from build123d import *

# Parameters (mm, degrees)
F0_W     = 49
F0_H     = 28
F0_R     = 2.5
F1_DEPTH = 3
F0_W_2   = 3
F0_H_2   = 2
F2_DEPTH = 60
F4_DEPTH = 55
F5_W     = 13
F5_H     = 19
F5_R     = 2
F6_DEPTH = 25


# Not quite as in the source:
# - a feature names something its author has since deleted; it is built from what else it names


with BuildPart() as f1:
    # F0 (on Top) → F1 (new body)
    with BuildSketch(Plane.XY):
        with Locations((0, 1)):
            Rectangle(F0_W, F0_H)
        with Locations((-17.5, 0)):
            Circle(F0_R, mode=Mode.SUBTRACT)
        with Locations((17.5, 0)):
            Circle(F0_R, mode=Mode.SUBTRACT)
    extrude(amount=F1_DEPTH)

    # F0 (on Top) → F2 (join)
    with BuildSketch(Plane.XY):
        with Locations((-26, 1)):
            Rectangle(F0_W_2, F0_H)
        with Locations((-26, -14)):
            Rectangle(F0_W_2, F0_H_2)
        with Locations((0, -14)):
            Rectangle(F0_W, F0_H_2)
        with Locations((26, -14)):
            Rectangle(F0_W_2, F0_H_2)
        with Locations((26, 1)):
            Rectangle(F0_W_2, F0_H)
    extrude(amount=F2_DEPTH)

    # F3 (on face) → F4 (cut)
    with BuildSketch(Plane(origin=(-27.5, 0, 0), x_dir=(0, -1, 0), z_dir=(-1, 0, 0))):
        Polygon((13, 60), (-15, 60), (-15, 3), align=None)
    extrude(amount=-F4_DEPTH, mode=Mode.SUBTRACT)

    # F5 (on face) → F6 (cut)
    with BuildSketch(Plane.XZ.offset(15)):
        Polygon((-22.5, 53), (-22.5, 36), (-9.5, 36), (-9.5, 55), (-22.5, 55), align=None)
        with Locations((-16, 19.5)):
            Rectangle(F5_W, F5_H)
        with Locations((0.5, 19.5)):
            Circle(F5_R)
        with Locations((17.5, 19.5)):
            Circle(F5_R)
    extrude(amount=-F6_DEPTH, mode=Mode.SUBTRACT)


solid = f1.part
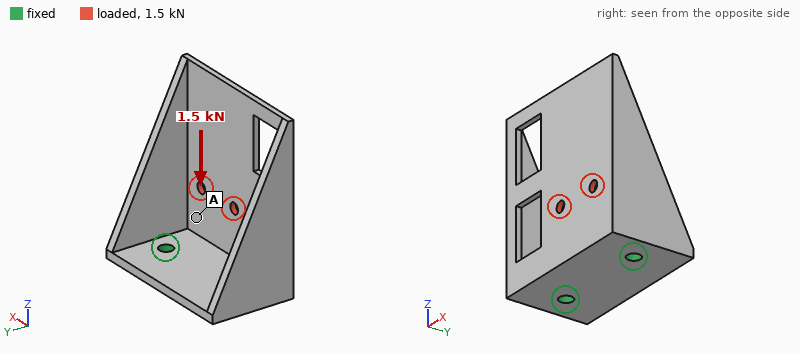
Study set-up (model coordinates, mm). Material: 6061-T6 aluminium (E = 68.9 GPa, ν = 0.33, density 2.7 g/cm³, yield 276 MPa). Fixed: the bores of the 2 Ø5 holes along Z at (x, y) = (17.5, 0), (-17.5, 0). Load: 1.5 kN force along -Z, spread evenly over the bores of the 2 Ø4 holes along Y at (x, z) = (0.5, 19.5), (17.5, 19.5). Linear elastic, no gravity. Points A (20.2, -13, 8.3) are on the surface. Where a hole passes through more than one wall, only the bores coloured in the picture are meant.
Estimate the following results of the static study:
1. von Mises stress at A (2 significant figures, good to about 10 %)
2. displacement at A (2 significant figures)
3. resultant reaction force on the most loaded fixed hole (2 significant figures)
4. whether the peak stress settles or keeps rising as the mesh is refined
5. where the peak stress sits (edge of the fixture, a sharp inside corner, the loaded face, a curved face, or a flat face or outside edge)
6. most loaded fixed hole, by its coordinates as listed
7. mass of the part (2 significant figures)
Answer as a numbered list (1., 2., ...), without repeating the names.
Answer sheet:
1. 29 MPa
2. 0.14 mm
3. 1.1 kN
4. keeps rising
5. edge of the fixture
6. (17.5, 0)
7. 40 g
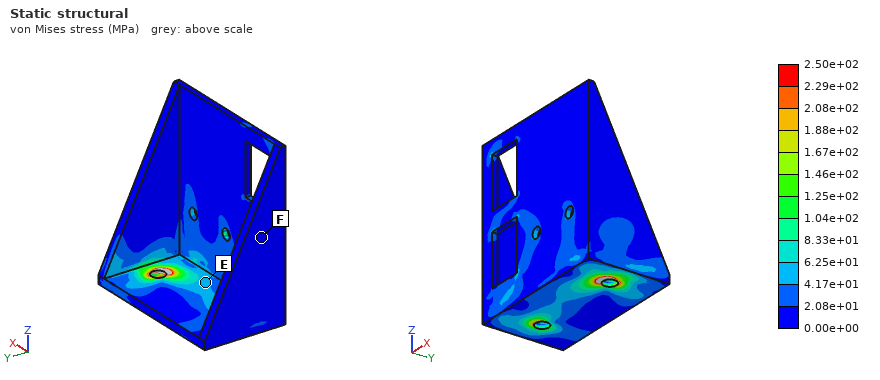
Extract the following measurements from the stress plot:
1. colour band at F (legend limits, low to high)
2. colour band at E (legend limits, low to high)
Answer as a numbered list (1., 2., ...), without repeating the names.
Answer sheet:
1. 0.00e+00 to 2.08e+01 MPa
2. 4.17e+01 to 6.25e+01 MPa
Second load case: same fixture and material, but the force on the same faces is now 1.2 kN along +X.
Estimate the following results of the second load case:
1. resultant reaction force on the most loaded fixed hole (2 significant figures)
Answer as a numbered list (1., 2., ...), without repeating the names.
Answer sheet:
1. 890 N
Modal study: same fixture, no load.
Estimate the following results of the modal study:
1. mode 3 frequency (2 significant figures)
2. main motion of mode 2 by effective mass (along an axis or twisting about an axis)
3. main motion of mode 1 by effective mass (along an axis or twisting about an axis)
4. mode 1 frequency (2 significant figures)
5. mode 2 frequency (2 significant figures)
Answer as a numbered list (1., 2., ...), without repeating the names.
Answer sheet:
1. 3600 Hz
2. along X
3. along Y
4. 1400 Hz
5. 1800 Hz
